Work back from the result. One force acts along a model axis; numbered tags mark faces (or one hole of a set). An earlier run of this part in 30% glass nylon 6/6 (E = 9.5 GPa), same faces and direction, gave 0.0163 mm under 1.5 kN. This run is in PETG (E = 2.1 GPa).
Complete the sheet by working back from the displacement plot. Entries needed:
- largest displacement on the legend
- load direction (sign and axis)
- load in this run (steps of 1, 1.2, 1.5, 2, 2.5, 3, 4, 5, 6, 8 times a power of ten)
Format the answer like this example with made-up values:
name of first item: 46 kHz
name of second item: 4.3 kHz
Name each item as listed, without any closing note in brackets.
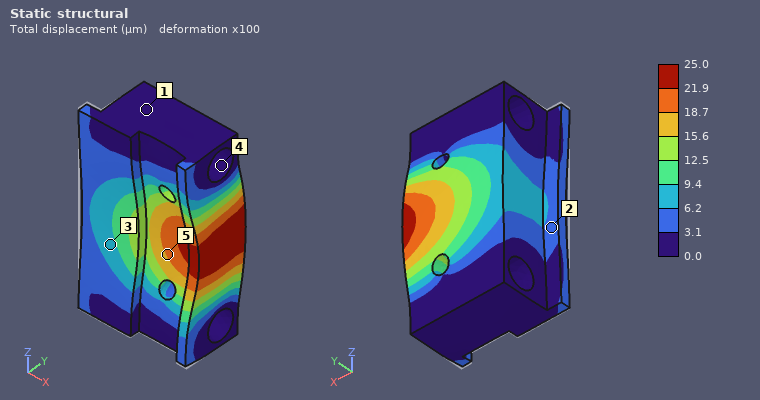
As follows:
largest displacement on the legend: 25.0 µm
load direction: +Y
load in this run: 500 N
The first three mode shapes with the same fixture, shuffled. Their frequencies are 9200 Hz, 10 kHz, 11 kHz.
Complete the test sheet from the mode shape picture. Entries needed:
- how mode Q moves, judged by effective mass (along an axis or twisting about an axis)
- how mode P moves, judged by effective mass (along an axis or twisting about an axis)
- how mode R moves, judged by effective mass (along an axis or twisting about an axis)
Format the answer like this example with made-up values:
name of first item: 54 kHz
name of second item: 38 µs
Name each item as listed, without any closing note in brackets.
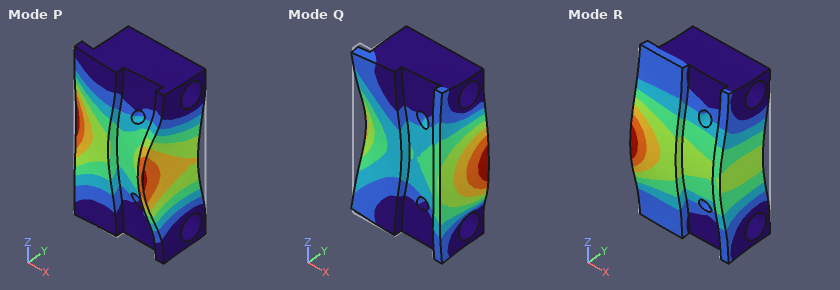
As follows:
how mode Q moves, judged by effective mass: along X
how mode P moves, judged by effective mass: along X
how mode R moves, judged by effective mass: along Y
